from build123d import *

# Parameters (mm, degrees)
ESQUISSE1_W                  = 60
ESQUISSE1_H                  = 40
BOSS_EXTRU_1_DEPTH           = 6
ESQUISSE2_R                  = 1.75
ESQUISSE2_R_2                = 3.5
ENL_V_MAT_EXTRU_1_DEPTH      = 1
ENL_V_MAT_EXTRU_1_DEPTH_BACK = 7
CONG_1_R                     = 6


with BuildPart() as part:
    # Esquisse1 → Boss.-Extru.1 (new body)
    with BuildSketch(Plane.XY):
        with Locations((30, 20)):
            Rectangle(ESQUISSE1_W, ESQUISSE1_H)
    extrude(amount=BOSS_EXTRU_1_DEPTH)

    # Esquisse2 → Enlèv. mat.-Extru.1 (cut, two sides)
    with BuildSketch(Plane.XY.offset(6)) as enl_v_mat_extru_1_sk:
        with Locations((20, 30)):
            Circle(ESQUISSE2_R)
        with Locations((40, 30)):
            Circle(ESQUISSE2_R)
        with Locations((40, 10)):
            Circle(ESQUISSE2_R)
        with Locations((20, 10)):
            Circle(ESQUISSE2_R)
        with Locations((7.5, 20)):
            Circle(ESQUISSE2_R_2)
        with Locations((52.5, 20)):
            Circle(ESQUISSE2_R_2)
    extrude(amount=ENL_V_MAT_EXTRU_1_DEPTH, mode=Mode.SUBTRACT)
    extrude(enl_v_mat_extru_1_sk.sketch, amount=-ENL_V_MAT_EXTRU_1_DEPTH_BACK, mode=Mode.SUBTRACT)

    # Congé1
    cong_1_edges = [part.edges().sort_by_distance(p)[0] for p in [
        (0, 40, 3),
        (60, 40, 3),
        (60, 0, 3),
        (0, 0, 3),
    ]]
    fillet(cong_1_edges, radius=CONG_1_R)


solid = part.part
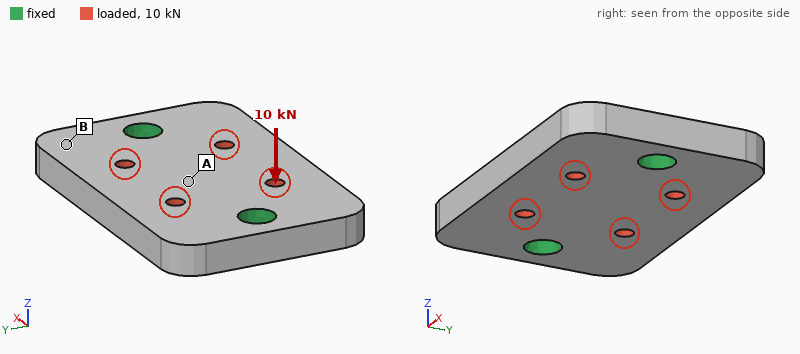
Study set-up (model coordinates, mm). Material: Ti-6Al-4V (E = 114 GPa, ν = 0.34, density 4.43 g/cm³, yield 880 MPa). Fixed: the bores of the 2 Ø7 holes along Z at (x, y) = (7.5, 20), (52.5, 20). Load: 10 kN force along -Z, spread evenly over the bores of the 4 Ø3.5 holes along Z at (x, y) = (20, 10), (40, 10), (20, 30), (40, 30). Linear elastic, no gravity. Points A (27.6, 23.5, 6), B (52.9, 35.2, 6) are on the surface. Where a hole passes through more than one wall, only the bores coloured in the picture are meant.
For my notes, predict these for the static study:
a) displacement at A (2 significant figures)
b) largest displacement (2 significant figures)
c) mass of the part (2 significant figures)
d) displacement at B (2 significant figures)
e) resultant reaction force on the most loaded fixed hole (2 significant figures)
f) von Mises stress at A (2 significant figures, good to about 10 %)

46 µm
72 µm
60 g
19 µm
5.0 kN
99 MPa
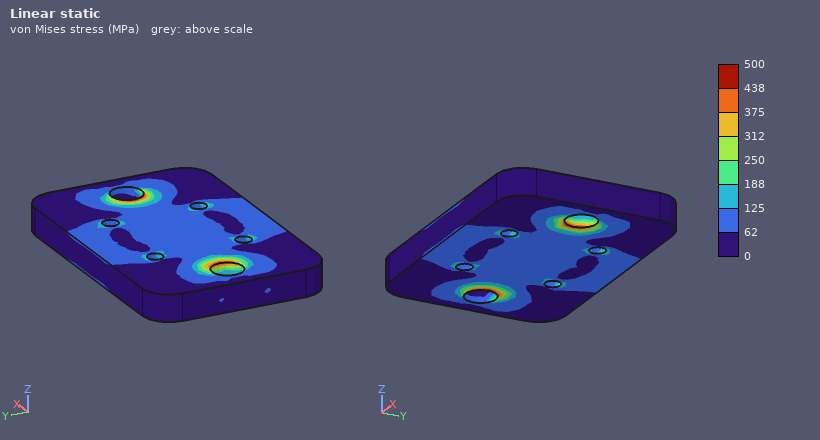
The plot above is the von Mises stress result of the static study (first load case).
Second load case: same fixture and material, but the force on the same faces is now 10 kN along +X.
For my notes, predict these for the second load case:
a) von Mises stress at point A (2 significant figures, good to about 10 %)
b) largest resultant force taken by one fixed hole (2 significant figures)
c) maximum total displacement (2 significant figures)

15 MPa
5.0 kN
6.9 µm
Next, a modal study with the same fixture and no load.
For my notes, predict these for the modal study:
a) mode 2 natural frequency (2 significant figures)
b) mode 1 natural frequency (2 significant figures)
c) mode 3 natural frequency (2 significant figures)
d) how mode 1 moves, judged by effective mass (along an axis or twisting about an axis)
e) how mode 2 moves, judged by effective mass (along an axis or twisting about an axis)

11 kHz
9200 Hz
16 kHz
twisting about X
along Z
